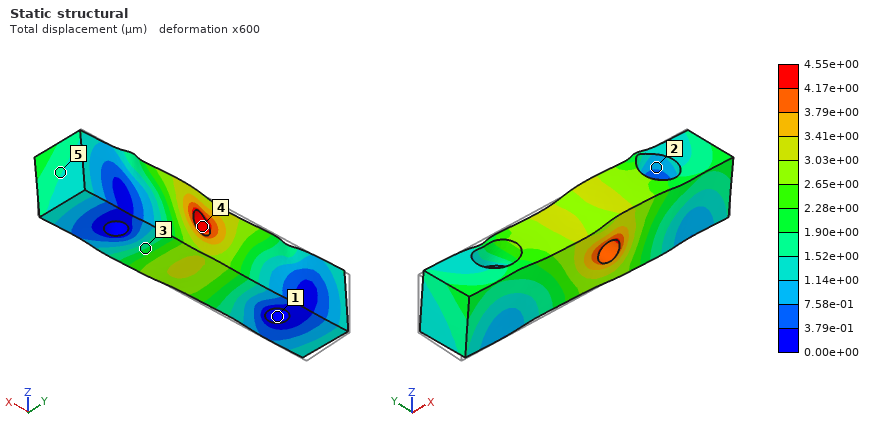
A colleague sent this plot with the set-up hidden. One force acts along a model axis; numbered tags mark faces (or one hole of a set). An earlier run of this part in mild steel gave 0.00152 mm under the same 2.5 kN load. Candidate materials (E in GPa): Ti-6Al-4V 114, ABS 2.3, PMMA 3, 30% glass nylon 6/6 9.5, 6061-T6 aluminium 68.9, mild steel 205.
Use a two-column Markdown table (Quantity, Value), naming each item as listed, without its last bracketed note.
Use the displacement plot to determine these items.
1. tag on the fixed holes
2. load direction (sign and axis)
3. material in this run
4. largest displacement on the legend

| Quantity | Value |
|---|---|
| tag on the fixed holes | 1 |
| load direction | +X |
| material in this run | 6061-T6 aluminium |
| largest displacement on the legend | 4.55e+00 µm |
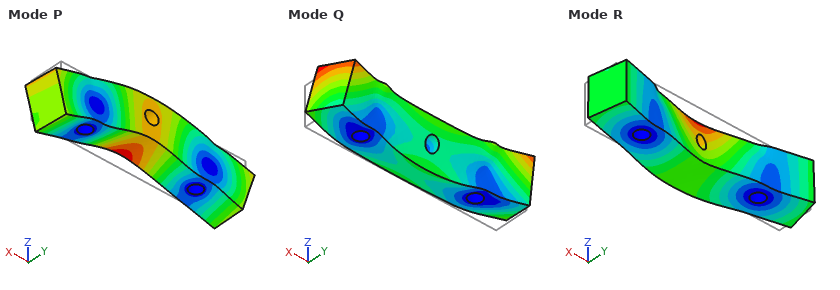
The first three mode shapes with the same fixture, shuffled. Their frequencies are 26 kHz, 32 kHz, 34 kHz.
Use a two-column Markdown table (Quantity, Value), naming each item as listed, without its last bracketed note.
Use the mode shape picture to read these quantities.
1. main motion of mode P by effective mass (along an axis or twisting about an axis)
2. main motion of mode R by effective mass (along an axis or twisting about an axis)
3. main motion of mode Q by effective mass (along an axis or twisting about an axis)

| Quantity | Value |
|---|---|
| main motion of mode P by effective mass | along Z |
| main motion of mode R by effective mass | along Y |
| main motion of mode Q by effective mass | along Y |
